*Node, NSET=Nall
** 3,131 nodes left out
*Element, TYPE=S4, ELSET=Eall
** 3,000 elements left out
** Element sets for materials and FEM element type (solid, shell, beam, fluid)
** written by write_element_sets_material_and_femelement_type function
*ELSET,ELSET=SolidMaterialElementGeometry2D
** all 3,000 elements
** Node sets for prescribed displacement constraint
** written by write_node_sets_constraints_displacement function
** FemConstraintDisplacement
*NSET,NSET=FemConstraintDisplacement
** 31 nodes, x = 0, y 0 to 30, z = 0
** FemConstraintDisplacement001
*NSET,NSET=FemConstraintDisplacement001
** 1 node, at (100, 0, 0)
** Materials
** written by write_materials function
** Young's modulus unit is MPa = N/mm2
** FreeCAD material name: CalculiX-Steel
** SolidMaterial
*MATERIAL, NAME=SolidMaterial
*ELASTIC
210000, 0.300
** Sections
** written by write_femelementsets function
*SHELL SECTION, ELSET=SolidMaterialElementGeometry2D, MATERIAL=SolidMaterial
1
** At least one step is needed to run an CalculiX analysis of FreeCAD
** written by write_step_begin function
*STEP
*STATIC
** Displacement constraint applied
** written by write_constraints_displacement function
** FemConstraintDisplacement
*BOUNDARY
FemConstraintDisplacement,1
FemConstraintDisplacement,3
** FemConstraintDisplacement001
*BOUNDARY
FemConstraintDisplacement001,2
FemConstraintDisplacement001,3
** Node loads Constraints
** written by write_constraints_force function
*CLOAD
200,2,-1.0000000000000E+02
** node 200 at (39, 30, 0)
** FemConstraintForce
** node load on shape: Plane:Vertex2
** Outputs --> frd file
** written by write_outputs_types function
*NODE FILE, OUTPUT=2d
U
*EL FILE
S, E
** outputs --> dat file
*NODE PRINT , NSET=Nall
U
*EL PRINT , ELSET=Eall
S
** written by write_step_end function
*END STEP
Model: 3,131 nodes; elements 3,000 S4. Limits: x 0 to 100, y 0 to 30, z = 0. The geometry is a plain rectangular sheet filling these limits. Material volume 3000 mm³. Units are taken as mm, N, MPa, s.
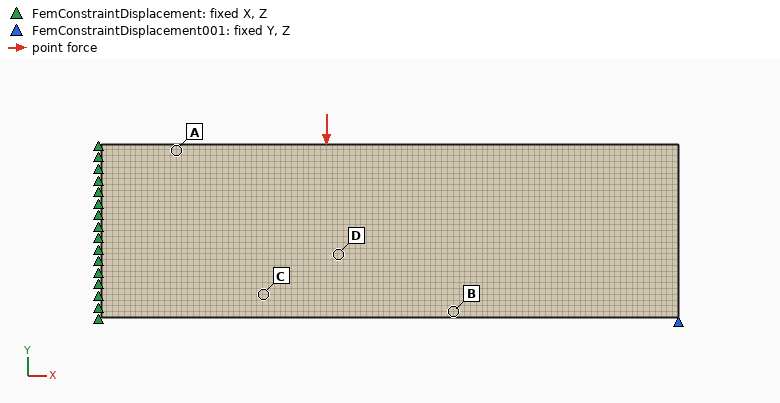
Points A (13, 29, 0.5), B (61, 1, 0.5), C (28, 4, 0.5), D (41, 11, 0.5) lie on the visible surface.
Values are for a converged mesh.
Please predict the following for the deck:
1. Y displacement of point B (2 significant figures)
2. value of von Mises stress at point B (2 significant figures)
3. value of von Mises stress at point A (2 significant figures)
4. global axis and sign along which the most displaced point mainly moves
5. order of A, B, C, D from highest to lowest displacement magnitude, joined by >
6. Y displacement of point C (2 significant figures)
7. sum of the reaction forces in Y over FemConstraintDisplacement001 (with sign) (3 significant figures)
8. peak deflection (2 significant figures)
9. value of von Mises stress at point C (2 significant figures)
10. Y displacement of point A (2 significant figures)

-0.039 mm
25 MPa
38 MPa
-Y
A > C > D > B
-0.059 mm
100 N
0.064 mm
30 MPa
-0.063 mm
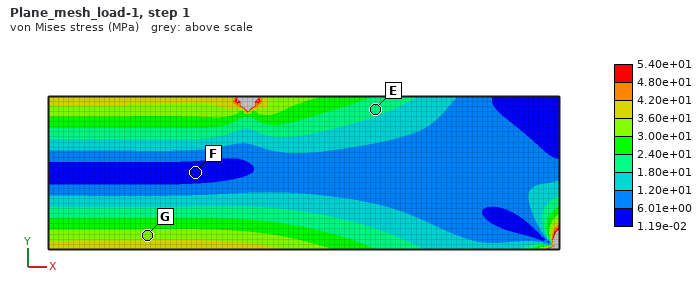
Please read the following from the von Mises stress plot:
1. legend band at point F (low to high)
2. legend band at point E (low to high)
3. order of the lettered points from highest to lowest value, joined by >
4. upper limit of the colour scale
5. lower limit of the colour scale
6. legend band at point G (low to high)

1.19e-02 to 6.01e+00 MPa
1.80e+01 to 2.40e+01 MPa
G > E > F
5.40e+01 MPa
1.19e-02 MPa
3.00e+01 to 3.60e+01 MPa
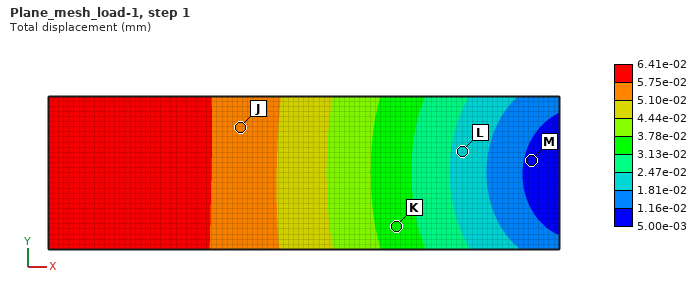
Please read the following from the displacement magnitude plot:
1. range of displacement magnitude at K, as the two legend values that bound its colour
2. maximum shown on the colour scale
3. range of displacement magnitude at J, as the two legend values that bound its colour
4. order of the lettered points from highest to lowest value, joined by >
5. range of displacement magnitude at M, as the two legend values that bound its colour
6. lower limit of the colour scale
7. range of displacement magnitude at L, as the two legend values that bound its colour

3.13e-02 to 3.78e-02 mm
6.41e-02 mm
5.10e-02 to 5.75e-02 mm
J > K > L > M
5.00e-03 to 1.16e-02 mm
5.00e-03 mm
1.81e-02 to 2.47e-02 mm
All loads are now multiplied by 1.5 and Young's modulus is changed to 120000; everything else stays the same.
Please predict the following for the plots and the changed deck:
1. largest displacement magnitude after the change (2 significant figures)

0.17 mm
